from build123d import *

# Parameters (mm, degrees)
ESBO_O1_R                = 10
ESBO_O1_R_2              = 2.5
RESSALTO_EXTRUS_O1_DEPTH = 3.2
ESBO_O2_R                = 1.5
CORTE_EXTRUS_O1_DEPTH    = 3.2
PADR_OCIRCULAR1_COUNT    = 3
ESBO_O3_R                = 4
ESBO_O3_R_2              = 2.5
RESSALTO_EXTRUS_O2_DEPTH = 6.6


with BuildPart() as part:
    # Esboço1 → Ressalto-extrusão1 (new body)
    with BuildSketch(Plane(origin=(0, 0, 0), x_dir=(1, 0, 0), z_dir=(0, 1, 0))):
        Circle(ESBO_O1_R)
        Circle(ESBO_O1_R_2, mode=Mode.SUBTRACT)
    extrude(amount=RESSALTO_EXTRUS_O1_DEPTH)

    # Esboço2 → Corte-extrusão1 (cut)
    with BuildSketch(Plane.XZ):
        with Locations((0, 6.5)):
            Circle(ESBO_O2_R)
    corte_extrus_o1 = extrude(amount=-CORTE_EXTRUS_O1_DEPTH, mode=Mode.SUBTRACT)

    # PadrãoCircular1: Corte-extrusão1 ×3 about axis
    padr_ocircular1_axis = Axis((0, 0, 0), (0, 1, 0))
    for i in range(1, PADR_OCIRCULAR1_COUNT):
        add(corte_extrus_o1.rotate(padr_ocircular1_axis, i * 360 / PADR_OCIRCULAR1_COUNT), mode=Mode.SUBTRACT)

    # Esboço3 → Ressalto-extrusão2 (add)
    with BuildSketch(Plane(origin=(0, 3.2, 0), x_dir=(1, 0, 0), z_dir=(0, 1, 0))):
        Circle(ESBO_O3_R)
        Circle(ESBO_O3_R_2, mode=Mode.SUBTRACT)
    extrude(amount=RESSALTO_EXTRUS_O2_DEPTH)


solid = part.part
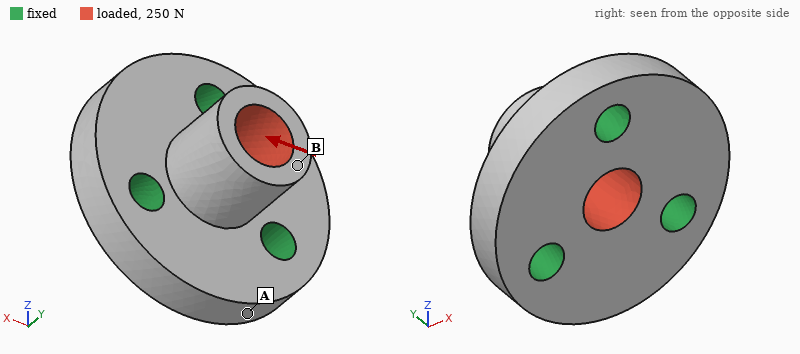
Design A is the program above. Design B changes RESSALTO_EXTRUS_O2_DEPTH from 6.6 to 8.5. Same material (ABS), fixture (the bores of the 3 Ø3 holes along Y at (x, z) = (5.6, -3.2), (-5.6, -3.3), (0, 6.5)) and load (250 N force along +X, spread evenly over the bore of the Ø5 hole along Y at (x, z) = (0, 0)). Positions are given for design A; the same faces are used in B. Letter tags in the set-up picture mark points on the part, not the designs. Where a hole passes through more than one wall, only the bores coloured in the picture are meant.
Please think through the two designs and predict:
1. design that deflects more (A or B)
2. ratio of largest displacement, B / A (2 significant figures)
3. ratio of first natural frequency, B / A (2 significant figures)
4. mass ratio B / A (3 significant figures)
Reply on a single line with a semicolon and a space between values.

B; 1.6; 0.76; 1.05
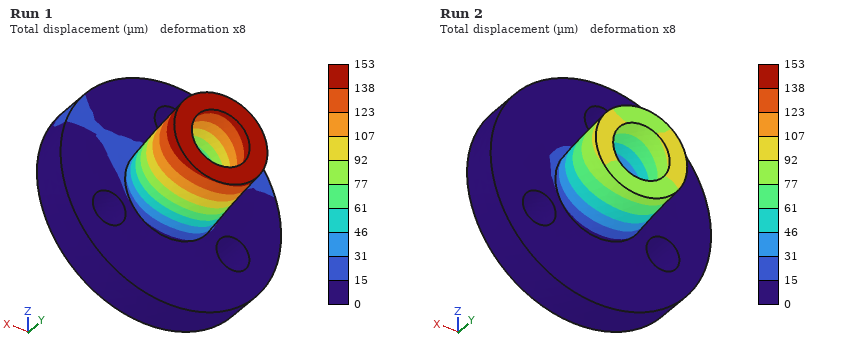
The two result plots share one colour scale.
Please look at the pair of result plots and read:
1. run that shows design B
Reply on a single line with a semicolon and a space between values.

Run 1
